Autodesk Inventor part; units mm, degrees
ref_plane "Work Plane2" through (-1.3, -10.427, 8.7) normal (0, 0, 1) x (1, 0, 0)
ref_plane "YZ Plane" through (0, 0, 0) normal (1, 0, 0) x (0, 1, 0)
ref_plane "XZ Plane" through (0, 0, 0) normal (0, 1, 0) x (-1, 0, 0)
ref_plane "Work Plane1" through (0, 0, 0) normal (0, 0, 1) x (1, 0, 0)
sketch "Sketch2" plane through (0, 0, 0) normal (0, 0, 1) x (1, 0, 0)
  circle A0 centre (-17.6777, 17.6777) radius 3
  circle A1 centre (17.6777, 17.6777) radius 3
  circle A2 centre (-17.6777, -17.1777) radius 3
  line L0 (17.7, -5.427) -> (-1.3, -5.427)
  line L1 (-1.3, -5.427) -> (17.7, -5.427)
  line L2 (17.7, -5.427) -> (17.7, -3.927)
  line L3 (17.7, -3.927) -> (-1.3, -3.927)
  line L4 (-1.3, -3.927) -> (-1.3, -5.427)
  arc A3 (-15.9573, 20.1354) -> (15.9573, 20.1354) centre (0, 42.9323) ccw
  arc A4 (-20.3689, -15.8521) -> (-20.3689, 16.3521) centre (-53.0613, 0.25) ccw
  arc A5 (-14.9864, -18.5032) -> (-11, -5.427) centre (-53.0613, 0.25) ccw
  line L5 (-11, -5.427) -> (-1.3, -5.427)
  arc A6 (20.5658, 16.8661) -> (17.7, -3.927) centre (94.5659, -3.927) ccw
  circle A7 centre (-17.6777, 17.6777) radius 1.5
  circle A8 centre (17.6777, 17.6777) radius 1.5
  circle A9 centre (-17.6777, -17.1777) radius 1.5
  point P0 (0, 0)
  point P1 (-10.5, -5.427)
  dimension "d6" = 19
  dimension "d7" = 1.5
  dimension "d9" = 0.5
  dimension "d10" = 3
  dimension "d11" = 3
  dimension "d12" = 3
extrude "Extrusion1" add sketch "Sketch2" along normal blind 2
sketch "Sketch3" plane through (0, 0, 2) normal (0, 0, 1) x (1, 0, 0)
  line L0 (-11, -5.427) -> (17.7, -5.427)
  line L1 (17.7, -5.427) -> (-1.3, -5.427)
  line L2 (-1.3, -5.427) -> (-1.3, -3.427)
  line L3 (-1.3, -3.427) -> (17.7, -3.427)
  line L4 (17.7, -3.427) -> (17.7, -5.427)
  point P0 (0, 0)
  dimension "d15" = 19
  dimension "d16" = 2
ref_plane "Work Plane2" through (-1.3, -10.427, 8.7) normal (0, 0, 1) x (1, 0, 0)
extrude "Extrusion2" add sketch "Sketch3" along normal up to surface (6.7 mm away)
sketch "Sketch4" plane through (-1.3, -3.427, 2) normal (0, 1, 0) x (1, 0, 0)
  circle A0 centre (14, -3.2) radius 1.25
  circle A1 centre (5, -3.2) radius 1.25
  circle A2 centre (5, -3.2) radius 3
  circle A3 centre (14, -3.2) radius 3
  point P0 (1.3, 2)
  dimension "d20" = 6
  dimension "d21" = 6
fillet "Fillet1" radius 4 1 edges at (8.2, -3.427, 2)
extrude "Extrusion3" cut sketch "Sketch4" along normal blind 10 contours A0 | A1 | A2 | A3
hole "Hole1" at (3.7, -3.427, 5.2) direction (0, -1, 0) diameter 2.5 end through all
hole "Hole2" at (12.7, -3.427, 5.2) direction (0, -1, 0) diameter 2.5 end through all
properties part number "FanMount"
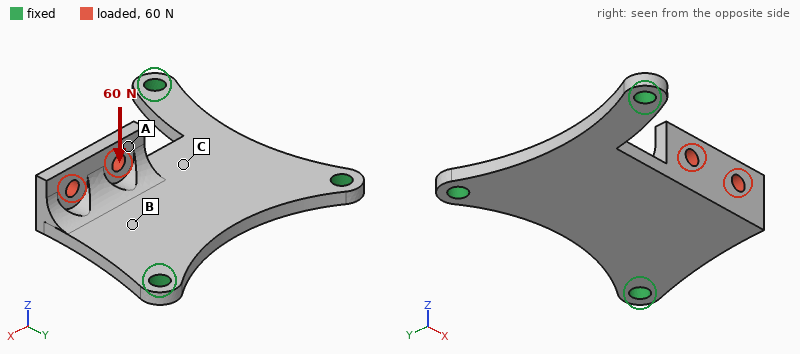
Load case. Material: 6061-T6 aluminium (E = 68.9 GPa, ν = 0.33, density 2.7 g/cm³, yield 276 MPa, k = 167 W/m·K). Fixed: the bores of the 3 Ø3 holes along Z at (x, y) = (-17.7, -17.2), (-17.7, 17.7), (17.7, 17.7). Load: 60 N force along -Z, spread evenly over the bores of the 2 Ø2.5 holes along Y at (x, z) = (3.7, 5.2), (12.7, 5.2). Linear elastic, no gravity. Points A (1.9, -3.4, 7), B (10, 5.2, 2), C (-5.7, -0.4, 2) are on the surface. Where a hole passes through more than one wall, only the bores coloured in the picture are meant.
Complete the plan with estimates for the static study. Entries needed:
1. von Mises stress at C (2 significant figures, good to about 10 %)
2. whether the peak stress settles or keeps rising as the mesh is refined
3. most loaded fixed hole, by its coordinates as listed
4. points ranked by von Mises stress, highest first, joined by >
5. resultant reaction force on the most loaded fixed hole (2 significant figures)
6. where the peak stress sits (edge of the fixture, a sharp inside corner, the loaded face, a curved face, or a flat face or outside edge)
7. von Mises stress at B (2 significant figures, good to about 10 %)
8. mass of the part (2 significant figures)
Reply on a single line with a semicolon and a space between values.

35 MPa; keeps rising; (17.7, 17.7); C > B > A; 40 N; edge of the fixture; 25 MPa; 5.6 g
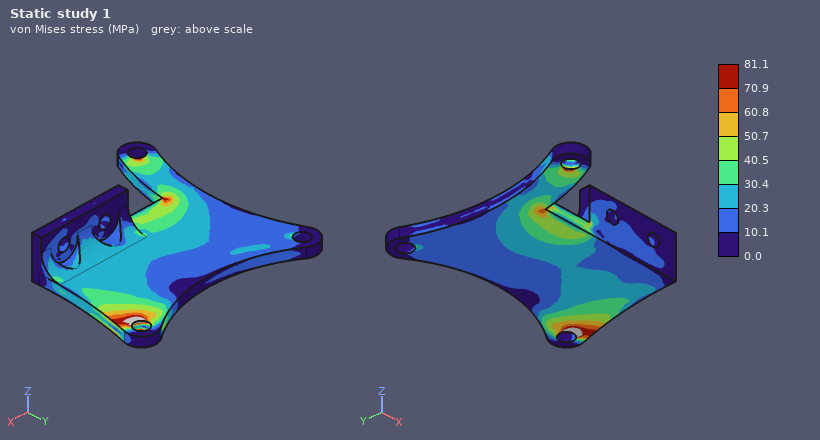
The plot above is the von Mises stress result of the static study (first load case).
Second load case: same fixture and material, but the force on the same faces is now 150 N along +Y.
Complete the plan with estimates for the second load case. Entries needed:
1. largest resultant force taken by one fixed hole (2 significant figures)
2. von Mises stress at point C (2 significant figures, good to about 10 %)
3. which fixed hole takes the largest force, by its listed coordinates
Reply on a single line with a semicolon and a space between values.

110 N; 32 MPa; (17.7, 17.7)
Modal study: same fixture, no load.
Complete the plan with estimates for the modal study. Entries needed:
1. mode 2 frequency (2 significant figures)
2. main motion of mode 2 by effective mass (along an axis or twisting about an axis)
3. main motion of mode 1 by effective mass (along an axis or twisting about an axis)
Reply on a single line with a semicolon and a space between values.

6600 Hz; along Z; along Z
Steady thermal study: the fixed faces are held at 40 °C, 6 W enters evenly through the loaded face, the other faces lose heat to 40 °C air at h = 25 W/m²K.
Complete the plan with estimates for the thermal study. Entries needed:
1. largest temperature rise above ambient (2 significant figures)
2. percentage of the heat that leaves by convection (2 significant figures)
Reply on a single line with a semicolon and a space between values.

20 K; 8.3 %
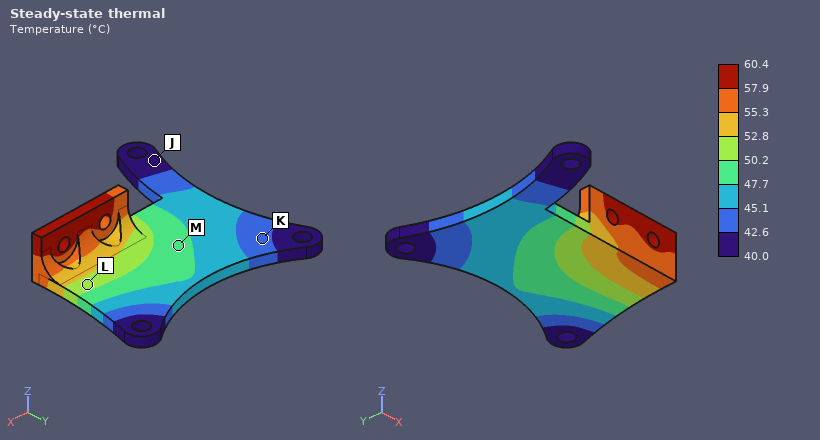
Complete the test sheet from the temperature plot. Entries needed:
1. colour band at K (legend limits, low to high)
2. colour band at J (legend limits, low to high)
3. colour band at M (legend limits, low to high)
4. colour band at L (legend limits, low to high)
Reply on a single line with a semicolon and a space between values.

42.6 to 45.1 °C; 40.0 to 42.6 °C; 47.7 to 50.2 °C; 50.2 to 52.8 °C
